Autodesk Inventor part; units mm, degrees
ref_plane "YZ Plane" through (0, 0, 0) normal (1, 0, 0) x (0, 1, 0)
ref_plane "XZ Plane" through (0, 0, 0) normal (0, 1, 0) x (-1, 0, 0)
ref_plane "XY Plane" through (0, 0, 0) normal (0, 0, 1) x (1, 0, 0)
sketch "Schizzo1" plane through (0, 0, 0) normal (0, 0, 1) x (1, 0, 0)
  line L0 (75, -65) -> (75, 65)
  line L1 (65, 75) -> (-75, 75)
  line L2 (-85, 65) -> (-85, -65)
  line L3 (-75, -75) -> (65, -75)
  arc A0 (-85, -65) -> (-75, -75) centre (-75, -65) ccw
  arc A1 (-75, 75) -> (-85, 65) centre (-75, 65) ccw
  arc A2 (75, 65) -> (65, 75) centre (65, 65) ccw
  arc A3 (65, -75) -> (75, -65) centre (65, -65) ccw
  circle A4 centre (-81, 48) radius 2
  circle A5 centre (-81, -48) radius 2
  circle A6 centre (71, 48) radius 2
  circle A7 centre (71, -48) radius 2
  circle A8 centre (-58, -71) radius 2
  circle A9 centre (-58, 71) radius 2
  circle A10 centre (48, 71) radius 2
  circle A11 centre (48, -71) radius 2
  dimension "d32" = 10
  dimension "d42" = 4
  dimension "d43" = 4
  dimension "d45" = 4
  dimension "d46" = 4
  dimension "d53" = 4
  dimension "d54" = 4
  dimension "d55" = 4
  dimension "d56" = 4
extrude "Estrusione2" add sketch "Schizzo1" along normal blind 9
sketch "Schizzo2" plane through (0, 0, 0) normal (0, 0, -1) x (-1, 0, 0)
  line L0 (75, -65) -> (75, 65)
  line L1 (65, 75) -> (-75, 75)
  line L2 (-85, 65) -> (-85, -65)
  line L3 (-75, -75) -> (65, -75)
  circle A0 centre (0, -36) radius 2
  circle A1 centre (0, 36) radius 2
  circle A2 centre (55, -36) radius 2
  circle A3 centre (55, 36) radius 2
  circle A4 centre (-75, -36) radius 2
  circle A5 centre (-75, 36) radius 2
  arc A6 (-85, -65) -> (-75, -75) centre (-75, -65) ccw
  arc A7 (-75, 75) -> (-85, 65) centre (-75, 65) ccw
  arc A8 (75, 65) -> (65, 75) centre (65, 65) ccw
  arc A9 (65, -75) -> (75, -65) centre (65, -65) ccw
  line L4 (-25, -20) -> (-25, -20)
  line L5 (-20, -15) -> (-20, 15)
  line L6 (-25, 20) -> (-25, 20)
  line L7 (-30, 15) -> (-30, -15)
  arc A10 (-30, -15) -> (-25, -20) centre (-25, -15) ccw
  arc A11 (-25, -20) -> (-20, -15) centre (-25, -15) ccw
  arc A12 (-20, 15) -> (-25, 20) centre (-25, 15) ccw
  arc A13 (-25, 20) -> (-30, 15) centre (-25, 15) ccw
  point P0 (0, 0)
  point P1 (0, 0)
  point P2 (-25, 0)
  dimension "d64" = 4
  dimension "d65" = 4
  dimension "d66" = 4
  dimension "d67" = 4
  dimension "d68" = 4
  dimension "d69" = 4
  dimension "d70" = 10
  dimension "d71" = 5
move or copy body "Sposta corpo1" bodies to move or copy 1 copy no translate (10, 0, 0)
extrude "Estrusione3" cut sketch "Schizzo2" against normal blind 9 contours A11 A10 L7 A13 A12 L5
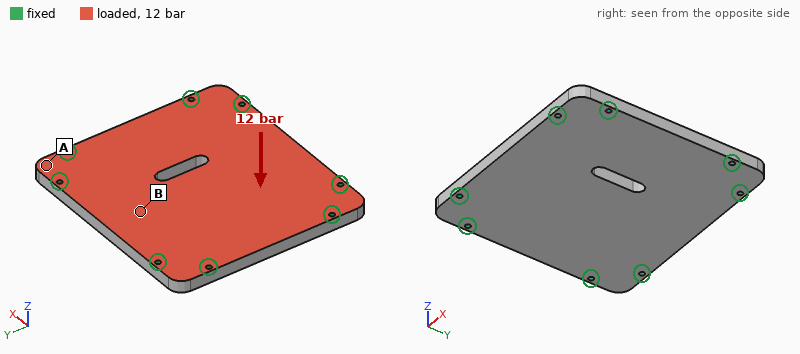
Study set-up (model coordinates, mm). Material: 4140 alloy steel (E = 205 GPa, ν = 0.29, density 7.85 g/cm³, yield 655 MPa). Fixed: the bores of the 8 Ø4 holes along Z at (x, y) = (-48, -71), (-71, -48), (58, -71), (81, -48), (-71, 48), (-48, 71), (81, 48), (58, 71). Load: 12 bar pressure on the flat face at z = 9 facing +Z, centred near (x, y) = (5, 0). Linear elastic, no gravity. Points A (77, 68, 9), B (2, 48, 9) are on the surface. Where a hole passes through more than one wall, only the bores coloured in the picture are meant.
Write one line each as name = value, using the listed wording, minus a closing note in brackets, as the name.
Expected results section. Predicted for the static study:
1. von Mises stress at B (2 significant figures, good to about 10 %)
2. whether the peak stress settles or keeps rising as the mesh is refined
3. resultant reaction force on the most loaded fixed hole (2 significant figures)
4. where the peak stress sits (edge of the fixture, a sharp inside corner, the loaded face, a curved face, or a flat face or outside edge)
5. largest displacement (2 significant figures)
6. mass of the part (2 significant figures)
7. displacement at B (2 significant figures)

von Mises stress at B = 69 MPa
whether the peak stress settles or keeps rising as the mesh is refined = keeps rising
resultant reaction force on the most loaded fixed hole = 3.9 kN
where the peak stress sits = edge of the fixture
largest displacement = 0.19 mm
mass of the part = 1.7 kg
displacement at B = 0.12 mm
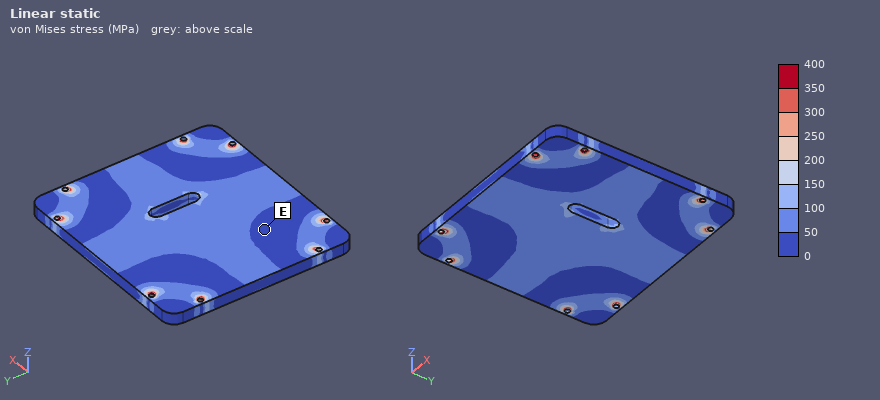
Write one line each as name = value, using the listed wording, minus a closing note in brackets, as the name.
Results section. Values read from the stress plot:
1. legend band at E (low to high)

legend band at E = 0 to 50 MPa
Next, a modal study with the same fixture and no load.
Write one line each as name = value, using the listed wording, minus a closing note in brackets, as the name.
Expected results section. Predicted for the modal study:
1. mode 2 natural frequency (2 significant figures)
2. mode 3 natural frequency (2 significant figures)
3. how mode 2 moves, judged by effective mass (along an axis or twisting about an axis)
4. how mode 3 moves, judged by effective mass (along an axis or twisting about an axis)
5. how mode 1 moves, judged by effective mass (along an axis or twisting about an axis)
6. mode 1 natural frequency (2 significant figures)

mode 2 natural frequency = 3600 Hz
mode 3 natural frequency = 3900 Hz
how mode 2 moves, judged by effective mass = twisting about X
how mode 3 moves, judged by effective mass = twisting about Y
how mode 1 moves, judged by effective mass = along Z
mode 1 natural frequency = 1900 Hz
